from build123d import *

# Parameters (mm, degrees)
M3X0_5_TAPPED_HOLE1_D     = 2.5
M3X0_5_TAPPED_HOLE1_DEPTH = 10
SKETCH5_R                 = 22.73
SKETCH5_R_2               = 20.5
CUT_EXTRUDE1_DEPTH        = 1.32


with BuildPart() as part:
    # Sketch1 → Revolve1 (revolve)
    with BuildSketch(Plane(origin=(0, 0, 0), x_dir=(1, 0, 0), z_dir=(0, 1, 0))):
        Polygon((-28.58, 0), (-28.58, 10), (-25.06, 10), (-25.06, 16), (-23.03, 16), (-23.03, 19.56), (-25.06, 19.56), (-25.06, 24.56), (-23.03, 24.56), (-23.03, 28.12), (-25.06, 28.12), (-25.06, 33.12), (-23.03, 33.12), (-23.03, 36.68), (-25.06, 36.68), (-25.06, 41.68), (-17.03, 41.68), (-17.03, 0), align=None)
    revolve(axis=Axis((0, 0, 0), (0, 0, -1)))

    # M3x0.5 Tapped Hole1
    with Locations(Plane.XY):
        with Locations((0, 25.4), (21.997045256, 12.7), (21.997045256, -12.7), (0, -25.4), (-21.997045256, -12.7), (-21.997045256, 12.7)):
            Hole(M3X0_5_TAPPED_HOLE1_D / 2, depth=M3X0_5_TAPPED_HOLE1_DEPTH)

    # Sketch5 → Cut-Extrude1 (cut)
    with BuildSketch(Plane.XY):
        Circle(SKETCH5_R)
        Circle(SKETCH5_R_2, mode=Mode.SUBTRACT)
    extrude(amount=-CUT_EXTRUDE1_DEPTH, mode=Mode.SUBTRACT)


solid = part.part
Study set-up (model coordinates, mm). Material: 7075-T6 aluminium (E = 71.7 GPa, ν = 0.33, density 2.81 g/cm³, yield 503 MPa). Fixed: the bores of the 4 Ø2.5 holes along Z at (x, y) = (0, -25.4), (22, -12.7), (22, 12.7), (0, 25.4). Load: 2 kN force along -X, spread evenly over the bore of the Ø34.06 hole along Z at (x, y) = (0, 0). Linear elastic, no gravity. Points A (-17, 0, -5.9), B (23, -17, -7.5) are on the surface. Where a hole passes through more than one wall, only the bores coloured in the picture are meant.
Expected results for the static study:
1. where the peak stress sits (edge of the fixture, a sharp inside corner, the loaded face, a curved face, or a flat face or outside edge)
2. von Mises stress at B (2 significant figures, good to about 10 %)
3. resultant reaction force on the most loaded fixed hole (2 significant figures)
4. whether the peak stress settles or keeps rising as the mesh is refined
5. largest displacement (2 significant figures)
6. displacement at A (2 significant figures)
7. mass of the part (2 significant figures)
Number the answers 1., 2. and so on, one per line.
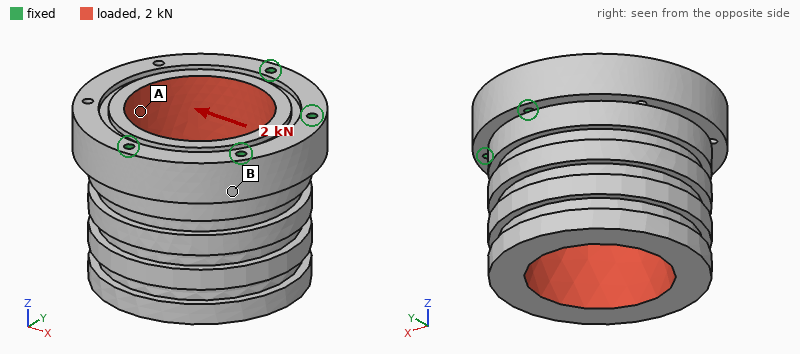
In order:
1. edge of the fixture
2. 5.5 MPa
3. 740 N
4. keeps rising
5. 15 µm
6. 6.2 µm
7. 130 g
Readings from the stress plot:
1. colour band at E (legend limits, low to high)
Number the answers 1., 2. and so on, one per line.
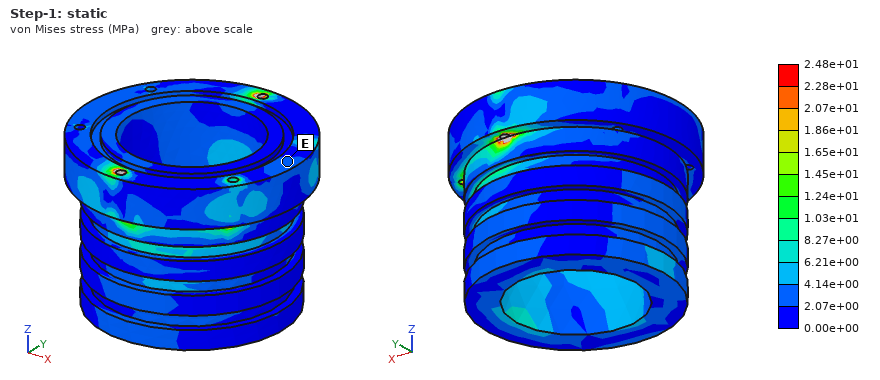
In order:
1. 2.07e+00 to 4.14e+00 MPa
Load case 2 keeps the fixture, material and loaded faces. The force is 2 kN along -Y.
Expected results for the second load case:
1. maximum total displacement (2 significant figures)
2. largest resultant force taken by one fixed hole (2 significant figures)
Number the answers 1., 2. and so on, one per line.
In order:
1. 5.4 µm
2. 870 N
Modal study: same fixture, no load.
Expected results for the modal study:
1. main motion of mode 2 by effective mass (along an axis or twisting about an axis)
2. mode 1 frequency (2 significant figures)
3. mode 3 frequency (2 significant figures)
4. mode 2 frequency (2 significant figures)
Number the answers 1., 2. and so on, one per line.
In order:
1. along Y
2. 5900 Hz
3. 13 kHz
4. 10 kHz
